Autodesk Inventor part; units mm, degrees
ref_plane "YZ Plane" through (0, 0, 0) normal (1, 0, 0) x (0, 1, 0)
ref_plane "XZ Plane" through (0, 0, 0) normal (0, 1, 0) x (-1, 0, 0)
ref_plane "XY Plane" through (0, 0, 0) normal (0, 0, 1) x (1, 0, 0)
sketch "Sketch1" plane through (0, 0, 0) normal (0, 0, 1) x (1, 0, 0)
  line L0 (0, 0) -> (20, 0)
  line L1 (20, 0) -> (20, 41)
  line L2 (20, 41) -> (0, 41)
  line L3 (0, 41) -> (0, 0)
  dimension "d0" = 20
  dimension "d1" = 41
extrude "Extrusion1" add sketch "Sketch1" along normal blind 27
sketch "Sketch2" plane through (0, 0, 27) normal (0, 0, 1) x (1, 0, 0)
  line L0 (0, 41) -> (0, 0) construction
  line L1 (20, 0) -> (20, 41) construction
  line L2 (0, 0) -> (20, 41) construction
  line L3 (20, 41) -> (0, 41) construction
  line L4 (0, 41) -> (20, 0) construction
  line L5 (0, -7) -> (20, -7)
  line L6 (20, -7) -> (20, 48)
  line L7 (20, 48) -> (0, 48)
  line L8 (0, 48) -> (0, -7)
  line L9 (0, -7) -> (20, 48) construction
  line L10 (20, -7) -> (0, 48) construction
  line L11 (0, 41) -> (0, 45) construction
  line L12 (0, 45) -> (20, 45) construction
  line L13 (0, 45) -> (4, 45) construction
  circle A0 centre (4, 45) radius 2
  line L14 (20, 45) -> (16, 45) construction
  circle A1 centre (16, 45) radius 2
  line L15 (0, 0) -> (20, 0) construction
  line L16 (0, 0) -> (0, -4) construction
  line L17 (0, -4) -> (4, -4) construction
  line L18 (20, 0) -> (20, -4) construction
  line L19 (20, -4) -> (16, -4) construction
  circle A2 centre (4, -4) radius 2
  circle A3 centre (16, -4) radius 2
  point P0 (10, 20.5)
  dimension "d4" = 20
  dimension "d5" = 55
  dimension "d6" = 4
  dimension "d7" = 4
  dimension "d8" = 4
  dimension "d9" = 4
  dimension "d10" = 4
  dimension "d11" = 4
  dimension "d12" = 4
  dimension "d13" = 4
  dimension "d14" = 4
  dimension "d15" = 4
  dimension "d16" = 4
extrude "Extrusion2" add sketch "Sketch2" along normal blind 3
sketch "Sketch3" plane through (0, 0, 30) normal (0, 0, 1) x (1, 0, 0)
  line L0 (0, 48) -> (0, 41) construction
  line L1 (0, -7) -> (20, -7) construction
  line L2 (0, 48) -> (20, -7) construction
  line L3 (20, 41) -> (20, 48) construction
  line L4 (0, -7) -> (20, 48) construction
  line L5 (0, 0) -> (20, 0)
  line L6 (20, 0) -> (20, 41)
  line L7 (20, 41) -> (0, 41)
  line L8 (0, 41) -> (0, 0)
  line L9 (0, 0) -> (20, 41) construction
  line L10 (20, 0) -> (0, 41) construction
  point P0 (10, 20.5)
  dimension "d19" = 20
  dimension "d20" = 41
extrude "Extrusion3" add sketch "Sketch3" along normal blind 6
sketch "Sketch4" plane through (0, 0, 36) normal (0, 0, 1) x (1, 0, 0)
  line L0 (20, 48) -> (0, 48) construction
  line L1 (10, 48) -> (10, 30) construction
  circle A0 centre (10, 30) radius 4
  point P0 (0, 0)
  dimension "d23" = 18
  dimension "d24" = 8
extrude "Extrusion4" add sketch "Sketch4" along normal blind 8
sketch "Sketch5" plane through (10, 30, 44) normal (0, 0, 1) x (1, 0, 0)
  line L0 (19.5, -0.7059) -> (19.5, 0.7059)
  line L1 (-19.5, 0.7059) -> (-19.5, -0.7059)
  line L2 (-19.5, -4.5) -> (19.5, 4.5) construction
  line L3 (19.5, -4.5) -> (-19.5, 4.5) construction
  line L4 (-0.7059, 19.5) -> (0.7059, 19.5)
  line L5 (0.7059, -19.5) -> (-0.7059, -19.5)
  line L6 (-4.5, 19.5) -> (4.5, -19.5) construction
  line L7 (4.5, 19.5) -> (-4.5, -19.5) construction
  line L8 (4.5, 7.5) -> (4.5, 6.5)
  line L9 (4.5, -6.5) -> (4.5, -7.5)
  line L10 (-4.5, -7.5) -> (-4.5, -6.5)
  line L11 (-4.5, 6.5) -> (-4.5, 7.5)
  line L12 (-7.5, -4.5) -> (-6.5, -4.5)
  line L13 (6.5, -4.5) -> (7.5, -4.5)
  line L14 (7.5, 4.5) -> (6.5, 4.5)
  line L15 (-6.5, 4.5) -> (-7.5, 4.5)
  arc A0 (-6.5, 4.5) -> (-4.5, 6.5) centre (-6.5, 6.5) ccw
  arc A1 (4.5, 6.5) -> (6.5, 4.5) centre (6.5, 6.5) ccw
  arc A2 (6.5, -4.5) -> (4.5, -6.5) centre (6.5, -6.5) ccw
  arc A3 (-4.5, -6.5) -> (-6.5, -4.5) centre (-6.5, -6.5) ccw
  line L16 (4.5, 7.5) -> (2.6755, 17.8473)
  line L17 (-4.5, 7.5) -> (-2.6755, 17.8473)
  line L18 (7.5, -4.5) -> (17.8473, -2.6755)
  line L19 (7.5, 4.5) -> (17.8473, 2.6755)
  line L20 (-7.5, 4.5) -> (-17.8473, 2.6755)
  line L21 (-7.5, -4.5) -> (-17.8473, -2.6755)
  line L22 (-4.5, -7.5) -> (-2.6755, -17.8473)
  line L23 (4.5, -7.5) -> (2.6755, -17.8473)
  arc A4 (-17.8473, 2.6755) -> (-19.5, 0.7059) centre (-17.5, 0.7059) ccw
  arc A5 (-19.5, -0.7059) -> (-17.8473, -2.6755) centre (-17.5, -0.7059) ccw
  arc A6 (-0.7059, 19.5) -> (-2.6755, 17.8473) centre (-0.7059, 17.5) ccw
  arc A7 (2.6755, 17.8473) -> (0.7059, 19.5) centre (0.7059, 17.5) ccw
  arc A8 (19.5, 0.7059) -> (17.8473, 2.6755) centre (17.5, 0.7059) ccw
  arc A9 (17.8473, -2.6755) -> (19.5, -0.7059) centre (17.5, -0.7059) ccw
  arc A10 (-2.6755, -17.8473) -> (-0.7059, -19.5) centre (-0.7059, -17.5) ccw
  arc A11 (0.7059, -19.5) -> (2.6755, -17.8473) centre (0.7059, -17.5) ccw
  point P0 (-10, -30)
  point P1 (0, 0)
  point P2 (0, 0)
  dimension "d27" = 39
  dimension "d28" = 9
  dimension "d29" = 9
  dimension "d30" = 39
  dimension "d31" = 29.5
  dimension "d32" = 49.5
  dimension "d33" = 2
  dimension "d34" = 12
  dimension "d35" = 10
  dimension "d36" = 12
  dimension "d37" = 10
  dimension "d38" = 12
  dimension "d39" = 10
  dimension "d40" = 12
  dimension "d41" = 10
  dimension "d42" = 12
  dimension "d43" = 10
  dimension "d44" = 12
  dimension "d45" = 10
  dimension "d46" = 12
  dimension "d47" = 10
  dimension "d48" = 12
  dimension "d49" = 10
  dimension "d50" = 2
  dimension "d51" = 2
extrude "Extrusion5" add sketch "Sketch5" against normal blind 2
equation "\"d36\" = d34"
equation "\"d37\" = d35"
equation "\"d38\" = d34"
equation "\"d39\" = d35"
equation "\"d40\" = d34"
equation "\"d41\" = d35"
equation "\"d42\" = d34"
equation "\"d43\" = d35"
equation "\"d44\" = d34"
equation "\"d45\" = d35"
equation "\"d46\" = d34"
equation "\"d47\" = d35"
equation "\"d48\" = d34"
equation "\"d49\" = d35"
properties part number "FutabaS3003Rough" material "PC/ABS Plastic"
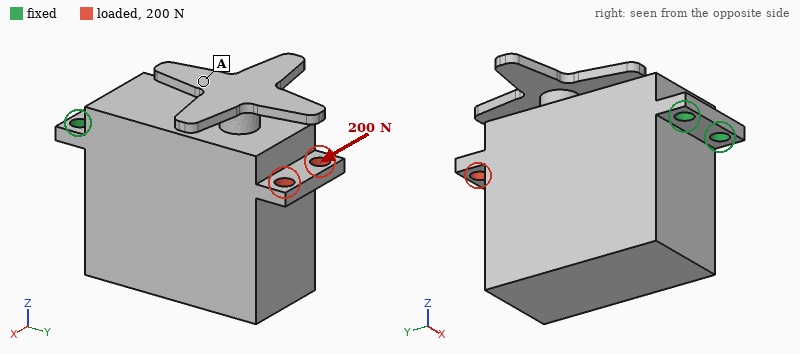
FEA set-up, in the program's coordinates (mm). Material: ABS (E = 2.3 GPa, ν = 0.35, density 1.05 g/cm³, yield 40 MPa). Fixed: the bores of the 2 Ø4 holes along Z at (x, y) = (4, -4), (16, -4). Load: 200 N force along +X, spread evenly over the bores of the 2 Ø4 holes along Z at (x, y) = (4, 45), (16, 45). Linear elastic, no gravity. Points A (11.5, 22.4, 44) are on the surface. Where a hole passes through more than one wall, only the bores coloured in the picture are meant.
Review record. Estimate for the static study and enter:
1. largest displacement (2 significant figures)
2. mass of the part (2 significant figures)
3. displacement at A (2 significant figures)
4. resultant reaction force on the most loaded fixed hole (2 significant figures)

0.88 mm
33 g
0.37 mm
710 N
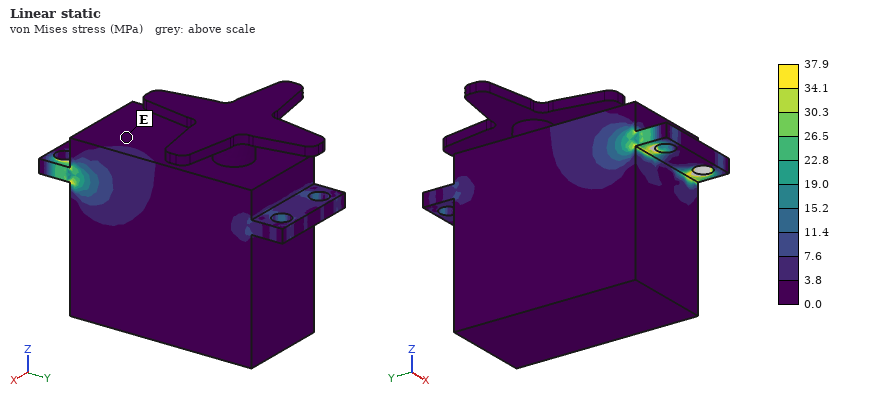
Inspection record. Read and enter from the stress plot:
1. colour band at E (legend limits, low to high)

0.0 to 3.8 MPa
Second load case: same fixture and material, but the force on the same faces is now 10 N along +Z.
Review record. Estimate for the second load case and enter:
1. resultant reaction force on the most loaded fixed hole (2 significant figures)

5.0 N
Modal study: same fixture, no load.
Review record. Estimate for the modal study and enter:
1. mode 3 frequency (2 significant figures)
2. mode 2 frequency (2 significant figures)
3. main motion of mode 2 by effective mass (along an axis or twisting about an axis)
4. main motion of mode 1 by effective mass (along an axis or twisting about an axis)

1100 Hz
710 Hz
along X
along Z
